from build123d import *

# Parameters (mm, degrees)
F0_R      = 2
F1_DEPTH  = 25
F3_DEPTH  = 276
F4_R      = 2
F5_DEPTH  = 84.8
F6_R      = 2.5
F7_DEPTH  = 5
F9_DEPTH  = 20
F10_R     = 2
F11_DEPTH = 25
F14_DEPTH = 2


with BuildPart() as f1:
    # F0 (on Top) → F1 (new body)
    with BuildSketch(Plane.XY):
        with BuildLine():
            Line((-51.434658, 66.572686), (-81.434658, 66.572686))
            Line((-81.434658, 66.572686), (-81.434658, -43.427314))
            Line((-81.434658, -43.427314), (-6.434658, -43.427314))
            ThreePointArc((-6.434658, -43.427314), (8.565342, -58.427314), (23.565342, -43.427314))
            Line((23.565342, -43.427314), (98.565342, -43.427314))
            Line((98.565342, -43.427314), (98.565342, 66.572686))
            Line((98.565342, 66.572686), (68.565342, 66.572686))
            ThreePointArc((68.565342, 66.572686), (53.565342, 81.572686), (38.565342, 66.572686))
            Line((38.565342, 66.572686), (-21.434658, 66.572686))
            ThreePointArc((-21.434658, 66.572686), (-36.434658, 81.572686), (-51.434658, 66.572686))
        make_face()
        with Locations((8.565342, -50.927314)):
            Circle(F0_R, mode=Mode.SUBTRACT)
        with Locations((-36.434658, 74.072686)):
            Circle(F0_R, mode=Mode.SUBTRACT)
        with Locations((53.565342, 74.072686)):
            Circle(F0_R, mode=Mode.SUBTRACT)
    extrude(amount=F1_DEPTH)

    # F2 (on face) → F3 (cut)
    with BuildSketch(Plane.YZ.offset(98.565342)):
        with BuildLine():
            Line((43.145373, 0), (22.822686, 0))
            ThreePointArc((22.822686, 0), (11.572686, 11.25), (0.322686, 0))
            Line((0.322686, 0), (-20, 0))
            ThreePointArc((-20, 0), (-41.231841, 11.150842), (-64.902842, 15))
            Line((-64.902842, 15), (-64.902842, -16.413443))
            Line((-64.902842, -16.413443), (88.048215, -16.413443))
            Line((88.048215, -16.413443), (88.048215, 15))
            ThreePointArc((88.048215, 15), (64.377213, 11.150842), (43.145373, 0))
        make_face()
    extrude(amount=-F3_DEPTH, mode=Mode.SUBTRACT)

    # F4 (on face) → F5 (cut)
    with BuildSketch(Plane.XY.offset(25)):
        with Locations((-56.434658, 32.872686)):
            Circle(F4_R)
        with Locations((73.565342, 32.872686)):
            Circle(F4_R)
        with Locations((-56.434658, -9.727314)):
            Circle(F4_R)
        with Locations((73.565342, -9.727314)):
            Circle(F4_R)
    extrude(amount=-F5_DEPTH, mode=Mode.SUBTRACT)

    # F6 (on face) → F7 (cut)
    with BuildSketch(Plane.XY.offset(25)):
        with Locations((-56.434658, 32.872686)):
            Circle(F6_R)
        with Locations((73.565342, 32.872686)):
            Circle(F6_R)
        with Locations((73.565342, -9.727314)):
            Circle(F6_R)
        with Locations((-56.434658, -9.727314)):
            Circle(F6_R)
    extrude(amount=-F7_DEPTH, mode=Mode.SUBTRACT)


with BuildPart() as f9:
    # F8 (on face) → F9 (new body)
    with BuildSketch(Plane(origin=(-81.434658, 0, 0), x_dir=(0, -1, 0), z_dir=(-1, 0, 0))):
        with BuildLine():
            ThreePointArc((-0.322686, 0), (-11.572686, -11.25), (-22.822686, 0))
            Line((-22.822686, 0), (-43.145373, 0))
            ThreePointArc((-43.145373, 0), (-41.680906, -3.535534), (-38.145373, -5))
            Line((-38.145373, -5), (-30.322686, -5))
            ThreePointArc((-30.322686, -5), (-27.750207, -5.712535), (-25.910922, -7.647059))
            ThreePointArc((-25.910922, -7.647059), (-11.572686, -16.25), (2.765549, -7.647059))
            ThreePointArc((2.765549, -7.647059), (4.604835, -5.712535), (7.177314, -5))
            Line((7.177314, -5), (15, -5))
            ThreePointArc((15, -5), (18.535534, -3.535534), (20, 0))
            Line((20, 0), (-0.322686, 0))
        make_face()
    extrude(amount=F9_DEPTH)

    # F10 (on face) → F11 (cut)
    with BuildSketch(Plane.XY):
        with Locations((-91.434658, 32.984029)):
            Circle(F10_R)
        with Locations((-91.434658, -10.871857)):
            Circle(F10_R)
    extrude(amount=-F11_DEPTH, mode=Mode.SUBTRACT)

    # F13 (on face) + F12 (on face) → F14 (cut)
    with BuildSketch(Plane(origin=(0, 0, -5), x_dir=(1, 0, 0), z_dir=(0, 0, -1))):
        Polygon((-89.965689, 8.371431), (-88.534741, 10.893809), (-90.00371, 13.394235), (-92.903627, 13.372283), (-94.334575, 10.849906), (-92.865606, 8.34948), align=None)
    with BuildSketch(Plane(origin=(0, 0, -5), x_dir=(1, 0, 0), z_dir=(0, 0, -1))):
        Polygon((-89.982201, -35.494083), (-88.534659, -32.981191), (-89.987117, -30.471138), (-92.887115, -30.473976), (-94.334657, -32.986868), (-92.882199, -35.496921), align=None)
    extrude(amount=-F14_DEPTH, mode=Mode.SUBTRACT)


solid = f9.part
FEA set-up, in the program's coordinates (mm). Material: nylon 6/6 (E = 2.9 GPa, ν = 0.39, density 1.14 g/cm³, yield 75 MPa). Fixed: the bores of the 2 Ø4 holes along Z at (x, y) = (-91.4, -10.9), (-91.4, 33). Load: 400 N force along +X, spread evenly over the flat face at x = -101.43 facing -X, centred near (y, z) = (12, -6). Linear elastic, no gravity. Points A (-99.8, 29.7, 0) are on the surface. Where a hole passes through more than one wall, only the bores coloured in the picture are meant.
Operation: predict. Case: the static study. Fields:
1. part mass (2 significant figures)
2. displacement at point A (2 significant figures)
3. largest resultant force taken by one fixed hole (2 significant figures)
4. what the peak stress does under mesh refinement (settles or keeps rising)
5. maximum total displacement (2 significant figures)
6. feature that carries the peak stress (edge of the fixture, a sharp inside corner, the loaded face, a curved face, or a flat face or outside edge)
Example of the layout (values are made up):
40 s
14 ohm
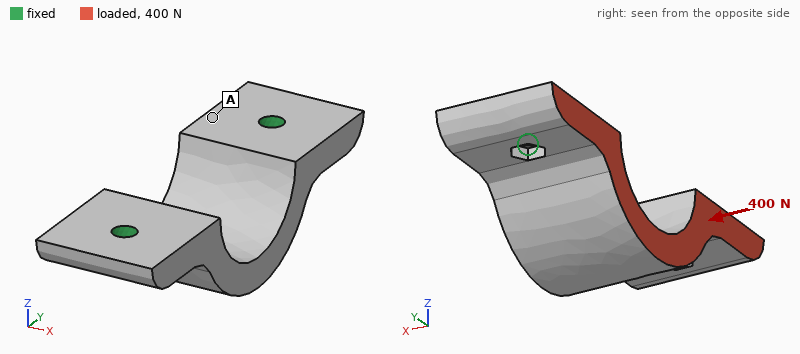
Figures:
8.1 g
0.099 mm
200 N
keeps rising
0.33 mm
edge of the fixture
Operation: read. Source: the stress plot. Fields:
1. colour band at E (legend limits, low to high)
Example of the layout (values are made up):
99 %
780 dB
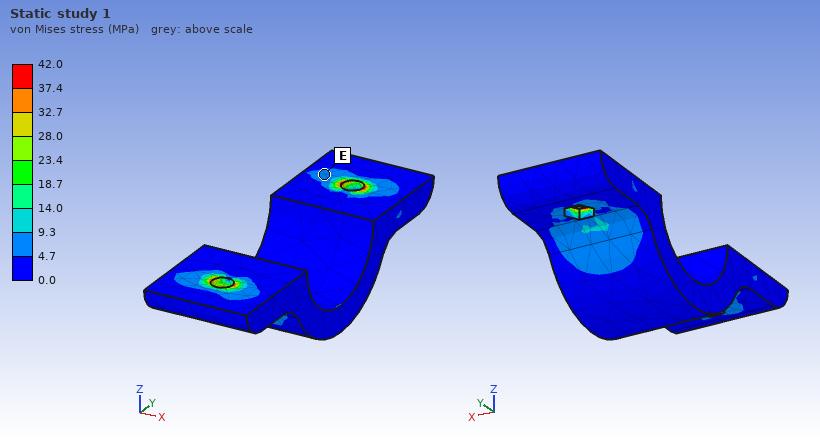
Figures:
4.7 to 9.3 MPa
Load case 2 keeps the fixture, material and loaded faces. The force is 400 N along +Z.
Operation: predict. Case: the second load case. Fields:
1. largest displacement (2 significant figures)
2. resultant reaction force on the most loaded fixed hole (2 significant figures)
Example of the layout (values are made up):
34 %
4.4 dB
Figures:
0.50 mm
230 N
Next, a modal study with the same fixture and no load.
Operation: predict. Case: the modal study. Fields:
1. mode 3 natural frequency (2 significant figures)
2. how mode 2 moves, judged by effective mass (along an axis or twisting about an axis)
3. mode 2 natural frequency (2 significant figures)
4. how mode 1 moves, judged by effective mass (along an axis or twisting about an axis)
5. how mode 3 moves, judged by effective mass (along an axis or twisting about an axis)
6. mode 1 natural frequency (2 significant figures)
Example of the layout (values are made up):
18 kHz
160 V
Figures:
5900 Hz
along Z
5400 Hz
along X
along Y
2200 Hz
